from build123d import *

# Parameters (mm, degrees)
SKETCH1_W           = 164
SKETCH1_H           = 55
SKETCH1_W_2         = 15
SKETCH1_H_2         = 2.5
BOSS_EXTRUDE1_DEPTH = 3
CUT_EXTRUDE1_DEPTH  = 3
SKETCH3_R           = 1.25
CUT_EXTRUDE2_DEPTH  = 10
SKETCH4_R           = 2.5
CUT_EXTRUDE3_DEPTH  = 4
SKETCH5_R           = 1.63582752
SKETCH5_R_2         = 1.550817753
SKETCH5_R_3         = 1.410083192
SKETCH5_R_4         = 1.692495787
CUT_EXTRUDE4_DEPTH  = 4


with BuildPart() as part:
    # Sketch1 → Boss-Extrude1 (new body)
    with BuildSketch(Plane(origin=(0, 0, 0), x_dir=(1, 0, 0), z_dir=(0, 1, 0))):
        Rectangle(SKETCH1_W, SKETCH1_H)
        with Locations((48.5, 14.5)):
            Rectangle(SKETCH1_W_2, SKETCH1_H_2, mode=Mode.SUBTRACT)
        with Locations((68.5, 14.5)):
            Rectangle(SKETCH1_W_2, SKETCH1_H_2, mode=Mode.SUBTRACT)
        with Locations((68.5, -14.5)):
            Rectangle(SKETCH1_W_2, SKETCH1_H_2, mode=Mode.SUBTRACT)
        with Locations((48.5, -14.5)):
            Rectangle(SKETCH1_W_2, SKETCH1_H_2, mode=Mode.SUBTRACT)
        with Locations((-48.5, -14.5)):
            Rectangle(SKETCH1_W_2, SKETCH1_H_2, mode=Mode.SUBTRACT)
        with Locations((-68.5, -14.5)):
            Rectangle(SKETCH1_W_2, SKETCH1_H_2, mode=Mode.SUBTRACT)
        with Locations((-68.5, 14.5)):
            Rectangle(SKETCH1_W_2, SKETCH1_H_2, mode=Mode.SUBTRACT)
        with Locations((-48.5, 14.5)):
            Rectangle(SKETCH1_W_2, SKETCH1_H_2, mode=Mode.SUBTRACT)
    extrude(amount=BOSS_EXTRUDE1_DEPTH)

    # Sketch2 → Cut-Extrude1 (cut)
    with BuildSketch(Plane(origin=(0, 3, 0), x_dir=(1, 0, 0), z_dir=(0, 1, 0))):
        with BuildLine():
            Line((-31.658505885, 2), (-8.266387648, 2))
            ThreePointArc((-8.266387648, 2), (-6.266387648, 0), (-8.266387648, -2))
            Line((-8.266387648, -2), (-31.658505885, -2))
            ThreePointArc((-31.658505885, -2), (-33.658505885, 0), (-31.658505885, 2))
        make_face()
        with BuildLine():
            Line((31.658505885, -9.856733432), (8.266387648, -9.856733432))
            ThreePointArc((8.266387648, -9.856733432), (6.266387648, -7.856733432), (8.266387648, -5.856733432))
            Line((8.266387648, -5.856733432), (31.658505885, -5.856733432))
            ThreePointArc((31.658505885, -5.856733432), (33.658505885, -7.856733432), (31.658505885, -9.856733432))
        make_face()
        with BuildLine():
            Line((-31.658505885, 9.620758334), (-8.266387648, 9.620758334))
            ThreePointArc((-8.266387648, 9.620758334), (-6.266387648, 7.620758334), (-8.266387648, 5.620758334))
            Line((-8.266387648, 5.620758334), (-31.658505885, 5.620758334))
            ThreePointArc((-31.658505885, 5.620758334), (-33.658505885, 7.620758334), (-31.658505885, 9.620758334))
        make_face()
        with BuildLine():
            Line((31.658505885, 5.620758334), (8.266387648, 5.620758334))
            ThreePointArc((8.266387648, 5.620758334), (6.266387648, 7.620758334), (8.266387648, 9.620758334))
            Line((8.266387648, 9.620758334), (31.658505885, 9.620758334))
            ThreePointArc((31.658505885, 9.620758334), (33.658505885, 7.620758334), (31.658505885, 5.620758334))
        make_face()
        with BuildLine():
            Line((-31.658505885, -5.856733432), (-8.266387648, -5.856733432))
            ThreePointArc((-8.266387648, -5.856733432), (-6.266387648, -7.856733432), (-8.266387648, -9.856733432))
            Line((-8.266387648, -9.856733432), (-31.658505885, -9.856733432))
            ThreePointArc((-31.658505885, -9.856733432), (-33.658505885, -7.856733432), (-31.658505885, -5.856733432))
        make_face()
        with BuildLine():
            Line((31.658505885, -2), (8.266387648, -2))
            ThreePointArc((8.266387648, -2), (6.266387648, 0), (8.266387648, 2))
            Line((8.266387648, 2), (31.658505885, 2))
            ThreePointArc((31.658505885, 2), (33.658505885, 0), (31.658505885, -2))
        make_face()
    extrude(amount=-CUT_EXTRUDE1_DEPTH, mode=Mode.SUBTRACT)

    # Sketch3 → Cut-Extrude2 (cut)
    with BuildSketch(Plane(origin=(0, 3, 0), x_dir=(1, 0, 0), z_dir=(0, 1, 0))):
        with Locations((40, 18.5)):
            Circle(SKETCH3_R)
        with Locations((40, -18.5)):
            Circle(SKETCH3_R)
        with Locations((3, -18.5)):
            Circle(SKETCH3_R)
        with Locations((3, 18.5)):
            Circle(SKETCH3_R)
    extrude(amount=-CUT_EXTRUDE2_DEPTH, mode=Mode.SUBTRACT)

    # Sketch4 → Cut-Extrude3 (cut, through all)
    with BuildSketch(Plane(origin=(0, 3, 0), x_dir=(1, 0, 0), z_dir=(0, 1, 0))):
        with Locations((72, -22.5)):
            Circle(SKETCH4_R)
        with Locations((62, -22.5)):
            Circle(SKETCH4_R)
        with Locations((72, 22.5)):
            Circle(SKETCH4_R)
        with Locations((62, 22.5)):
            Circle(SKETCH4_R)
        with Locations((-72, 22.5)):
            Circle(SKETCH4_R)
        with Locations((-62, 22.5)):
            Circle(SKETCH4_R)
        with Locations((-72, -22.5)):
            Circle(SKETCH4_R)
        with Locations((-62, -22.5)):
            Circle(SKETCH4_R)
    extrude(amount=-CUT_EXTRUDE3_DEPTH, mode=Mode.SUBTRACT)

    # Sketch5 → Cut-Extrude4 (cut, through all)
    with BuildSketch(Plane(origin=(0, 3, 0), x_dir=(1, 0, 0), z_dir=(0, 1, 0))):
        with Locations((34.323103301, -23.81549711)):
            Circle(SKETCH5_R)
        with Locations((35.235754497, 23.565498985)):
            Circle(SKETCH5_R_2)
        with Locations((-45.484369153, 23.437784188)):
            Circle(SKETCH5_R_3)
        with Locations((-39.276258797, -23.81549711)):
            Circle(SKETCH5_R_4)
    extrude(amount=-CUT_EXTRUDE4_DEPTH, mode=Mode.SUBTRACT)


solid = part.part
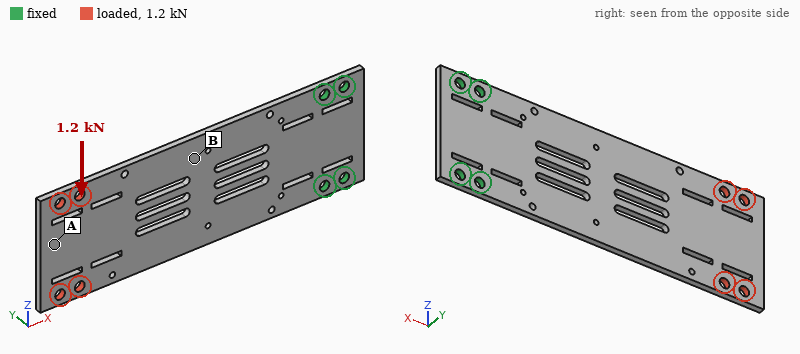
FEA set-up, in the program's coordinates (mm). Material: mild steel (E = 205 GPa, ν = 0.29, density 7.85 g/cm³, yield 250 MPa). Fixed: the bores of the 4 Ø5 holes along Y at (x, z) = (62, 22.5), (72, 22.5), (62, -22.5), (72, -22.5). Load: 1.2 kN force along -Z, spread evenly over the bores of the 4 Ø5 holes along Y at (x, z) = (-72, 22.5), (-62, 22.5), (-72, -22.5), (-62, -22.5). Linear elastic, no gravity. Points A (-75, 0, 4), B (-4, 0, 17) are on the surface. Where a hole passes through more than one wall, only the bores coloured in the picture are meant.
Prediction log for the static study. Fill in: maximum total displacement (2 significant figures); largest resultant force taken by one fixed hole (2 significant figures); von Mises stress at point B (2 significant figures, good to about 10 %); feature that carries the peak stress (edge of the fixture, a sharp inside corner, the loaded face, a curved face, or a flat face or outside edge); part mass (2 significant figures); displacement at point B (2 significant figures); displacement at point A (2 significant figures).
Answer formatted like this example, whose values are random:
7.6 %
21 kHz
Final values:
0.19 mm
3.1 kN
43 MPa
a curved face
190 g
0.066 mm
0.17 mm
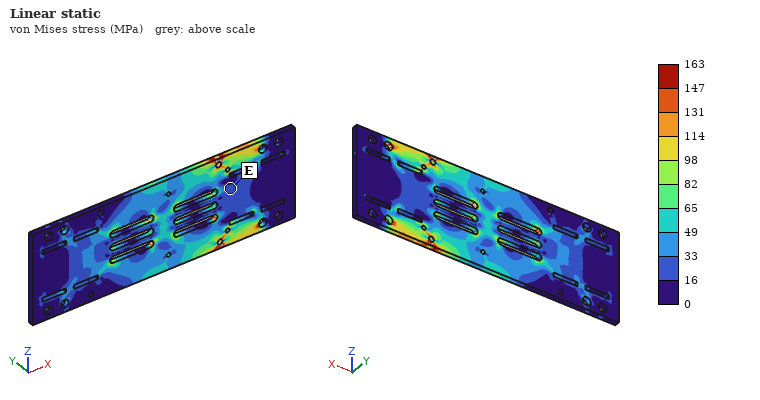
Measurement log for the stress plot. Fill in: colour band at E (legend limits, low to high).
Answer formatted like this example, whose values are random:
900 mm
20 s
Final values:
16 to 33 MPa
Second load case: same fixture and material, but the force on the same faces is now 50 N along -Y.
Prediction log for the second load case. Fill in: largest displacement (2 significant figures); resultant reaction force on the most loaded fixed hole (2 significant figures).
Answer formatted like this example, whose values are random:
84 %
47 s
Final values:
2.0 mm
110 N
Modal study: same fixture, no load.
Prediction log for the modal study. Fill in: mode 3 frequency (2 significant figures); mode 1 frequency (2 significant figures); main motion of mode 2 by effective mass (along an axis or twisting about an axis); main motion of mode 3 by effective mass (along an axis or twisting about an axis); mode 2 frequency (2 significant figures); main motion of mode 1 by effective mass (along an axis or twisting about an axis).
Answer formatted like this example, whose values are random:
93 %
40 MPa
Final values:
730 Hz
120 Hz
twisting about X
along Y
610 Hz
along Y
